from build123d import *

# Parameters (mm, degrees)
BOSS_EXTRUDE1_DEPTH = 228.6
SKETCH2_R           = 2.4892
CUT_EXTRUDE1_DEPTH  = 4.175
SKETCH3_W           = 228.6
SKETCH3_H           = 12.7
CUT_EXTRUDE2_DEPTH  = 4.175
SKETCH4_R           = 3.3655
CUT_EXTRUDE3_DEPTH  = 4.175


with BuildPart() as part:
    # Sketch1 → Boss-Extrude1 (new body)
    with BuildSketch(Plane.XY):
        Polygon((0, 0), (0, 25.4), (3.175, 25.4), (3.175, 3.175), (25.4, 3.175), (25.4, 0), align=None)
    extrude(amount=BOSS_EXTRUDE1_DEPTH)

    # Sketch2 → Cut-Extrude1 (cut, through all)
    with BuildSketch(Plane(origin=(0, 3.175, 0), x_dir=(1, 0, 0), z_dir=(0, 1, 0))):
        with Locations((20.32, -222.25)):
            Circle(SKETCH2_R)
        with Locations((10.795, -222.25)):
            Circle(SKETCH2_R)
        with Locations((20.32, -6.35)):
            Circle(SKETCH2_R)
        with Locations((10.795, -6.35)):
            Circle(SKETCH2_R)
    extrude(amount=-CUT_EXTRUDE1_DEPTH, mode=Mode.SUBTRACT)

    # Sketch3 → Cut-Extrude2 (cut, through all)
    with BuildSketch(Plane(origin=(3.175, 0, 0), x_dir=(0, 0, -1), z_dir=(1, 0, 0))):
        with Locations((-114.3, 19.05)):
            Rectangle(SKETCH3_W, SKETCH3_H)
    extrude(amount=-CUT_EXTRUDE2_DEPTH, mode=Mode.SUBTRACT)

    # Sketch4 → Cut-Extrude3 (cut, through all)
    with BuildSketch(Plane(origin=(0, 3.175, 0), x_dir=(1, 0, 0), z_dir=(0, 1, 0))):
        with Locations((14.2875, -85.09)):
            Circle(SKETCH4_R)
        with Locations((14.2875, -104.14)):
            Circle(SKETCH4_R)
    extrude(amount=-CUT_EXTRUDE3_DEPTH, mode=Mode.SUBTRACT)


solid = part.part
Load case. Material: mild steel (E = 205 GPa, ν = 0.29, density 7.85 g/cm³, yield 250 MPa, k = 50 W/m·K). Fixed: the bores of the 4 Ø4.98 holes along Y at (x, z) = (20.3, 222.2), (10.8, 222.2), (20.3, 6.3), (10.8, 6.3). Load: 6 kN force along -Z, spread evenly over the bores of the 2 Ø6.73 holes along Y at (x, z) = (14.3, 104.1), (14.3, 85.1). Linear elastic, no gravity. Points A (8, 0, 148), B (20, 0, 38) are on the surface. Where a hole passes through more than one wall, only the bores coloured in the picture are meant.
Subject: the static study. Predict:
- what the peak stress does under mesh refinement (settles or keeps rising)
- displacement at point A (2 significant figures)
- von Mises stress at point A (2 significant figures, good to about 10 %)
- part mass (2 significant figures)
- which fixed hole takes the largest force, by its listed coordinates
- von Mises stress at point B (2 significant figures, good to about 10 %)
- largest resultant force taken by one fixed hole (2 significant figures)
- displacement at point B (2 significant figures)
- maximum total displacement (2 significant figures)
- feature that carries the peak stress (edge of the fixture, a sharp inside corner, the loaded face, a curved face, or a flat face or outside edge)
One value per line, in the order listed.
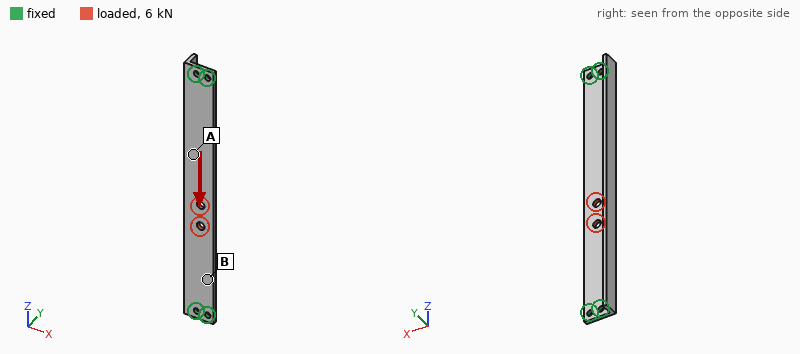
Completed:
keeps rising
22 µm
28 MPa
200 g
(10.8, 6.3)
50 MPa
2.5 kN
10 µm
24 µm
edge of the fixture
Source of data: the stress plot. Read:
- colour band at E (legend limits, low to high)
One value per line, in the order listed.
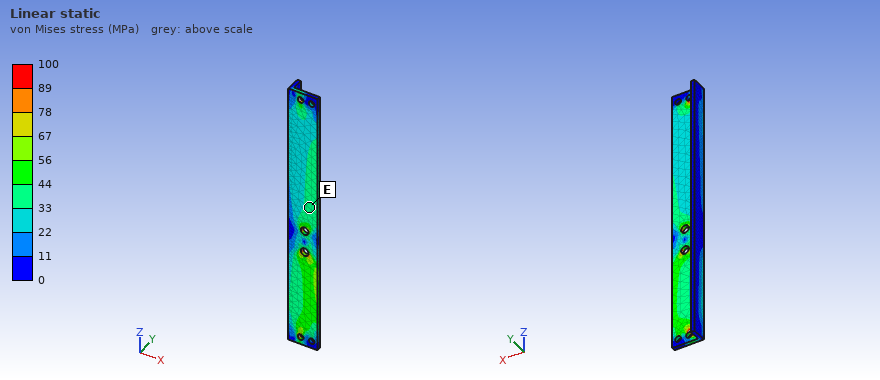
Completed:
33 to 44 MPa
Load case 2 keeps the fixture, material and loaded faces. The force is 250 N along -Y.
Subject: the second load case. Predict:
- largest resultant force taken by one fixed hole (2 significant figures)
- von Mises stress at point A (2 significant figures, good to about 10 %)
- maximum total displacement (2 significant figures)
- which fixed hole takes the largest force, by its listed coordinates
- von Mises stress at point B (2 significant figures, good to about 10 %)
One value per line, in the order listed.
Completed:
550 N
19 MPa
0.20 mm
(10.8, 6.3)
27 MPa
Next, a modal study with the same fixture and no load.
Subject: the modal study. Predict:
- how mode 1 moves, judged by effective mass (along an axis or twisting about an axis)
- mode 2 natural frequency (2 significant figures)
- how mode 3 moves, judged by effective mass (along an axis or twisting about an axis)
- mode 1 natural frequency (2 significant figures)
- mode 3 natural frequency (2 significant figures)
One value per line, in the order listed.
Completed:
along Y
1600 Hz
twisting about X
740 Hz
2000 Hz
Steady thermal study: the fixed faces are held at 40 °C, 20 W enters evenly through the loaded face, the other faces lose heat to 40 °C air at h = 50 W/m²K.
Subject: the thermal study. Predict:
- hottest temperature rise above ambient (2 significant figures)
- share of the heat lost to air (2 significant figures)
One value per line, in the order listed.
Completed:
70 K
87 %
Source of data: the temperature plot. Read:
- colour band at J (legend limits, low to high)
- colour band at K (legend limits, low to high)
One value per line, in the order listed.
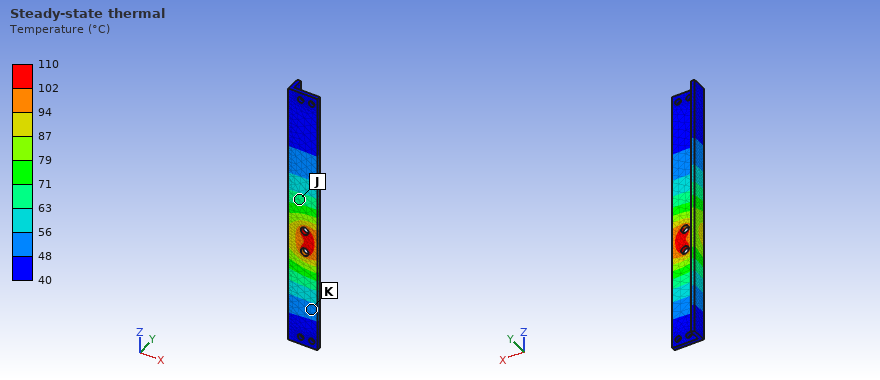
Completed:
63 to 71 °C
48 to 56 °C
